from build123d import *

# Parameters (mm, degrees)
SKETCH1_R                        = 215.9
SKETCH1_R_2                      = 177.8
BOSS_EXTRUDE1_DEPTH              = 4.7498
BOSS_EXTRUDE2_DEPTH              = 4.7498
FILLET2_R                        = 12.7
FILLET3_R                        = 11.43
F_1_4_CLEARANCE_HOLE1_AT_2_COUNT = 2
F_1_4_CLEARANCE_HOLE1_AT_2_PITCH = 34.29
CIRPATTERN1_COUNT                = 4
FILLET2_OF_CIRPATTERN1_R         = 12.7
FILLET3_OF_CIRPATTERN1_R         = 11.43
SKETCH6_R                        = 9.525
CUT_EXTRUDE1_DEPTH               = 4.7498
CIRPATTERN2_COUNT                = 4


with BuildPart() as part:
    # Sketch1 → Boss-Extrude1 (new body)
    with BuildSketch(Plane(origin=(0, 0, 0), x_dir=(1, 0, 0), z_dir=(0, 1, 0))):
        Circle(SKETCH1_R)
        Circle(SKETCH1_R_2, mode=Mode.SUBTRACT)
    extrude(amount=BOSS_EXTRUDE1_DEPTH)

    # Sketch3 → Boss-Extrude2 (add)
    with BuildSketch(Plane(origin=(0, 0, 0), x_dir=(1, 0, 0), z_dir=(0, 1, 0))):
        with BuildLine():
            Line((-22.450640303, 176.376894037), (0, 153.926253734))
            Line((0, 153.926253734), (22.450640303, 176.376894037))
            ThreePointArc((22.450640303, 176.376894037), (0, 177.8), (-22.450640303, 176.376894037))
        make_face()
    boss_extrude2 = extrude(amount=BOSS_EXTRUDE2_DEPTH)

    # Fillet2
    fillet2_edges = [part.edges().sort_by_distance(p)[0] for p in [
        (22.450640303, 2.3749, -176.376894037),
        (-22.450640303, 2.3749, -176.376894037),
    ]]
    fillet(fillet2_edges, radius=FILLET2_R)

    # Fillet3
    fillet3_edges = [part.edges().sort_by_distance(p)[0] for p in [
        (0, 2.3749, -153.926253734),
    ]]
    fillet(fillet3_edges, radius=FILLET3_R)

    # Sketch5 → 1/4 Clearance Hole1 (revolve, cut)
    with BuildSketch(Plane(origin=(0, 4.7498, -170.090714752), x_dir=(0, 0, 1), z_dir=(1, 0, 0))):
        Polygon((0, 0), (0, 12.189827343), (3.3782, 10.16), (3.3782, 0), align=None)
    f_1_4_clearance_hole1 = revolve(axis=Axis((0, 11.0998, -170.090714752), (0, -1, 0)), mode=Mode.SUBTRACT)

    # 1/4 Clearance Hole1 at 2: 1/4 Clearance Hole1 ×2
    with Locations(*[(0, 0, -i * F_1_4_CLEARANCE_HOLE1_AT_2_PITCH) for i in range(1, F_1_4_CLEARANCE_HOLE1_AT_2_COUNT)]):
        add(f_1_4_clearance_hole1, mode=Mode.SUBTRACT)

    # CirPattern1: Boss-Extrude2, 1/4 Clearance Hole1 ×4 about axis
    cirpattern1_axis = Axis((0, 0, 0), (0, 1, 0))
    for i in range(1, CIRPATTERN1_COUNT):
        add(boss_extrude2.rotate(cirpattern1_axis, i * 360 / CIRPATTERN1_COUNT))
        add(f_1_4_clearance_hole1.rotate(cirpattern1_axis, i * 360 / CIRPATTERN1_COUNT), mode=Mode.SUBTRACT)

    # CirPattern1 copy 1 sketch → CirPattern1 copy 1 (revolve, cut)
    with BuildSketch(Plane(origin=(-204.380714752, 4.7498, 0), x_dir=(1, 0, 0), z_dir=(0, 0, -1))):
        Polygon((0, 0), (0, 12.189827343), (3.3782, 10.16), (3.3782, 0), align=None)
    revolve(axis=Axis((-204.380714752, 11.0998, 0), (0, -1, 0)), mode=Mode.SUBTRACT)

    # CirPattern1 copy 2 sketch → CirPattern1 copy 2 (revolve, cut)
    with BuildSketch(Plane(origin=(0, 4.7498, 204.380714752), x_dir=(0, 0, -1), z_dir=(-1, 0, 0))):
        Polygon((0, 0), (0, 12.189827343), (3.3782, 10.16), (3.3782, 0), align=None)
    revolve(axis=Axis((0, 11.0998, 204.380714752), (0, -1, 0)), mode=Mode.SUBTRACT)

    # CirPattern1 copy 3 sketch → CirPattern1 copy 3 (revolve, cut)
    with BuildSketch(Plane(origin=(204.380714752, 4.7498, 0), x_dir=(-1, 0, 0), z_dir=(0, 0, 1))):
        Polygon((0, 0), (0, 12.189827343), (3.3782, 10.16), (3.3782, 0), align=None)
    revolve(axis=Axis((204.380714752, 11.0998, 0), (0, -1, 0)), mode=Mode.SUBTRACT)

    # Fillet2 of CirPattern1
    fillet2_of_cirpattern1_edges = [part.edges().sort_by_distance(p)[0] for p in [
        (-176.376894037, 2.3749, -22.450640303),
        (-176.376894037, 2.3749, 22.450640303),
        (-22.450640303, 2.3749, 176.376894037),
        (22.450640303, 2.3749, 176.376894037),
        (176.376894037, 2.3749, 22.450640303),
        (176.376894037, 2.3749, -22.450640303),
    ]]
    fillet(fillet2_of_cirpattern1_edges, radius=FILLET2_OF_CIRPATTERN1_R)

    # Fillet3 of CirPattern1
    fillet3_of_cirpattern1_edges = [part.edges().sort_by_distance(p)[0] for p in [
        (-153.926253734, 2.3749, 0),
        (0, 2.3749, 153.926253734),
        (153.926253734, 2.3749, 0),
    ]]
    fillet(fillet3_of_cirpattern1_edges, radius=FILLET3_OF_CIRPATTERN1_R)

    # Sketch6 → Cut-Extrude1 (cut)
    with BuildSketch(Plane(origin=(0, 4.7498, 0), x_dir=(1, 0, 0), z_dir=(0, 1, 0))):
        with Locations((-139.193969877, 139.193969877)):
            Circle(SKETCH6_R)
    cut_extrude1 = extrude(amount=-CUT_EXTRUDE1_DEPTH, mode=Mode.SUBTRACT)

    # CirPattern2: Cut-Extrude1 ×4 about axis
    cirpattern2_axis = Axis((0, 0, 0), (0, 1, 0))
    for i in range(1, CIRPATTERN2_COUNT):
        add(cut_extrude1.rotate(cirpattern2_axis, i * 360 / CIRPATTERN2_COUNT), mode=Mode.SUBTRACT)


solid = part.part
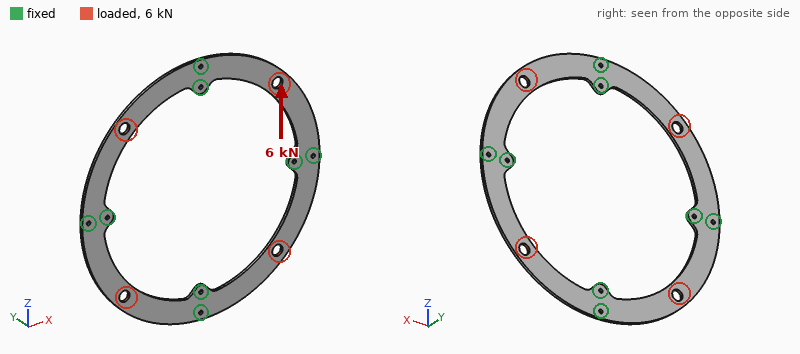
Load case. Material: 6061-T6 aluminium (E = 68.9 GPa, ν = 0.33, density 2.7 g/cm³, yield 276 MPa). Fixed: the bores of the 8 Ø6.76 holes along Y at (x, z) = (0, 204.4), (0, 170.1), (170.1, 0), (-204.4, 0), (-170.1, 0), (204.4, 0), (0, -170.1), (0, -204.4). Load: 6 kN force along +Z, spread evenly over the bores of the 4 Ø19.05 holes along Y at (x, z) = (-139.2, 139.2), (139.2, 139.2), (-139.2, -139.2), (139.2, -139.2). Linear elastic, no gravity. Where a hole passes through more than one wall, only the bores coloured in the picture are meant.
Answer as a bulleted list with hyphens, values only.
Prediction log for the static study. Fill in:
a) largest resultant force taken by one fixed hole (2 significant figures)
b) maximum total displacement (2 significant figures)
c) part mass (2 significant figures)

- 2.2 kN
- 46 µm
- 610 g
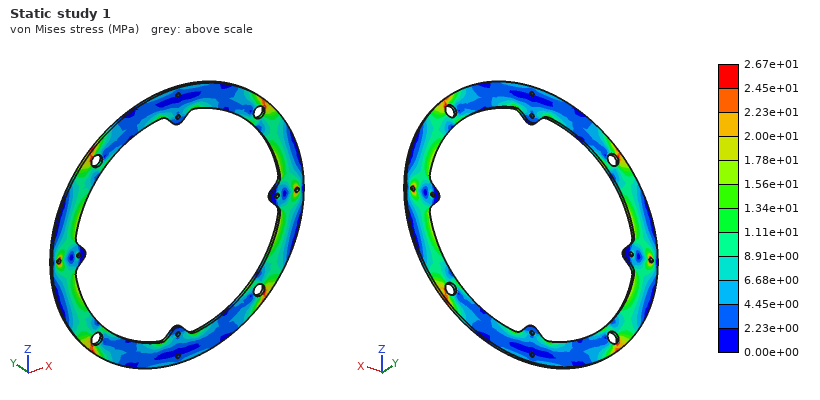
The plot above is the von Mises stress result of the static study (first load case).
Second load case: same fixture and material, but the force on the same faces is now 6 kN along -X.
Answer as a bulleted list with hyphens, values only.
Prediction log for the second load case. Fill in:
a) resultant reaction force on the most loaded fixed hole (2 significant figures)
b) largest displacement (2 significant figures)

- 2.2 kN
- 46 µm
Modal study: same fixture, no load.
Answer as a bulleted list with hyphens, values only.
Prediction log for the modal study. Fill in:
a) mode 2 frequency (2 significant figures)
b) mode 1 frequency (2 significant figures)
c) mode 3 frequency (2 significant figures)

- 250 Hz
- 250 Hz
- 250 Hz
